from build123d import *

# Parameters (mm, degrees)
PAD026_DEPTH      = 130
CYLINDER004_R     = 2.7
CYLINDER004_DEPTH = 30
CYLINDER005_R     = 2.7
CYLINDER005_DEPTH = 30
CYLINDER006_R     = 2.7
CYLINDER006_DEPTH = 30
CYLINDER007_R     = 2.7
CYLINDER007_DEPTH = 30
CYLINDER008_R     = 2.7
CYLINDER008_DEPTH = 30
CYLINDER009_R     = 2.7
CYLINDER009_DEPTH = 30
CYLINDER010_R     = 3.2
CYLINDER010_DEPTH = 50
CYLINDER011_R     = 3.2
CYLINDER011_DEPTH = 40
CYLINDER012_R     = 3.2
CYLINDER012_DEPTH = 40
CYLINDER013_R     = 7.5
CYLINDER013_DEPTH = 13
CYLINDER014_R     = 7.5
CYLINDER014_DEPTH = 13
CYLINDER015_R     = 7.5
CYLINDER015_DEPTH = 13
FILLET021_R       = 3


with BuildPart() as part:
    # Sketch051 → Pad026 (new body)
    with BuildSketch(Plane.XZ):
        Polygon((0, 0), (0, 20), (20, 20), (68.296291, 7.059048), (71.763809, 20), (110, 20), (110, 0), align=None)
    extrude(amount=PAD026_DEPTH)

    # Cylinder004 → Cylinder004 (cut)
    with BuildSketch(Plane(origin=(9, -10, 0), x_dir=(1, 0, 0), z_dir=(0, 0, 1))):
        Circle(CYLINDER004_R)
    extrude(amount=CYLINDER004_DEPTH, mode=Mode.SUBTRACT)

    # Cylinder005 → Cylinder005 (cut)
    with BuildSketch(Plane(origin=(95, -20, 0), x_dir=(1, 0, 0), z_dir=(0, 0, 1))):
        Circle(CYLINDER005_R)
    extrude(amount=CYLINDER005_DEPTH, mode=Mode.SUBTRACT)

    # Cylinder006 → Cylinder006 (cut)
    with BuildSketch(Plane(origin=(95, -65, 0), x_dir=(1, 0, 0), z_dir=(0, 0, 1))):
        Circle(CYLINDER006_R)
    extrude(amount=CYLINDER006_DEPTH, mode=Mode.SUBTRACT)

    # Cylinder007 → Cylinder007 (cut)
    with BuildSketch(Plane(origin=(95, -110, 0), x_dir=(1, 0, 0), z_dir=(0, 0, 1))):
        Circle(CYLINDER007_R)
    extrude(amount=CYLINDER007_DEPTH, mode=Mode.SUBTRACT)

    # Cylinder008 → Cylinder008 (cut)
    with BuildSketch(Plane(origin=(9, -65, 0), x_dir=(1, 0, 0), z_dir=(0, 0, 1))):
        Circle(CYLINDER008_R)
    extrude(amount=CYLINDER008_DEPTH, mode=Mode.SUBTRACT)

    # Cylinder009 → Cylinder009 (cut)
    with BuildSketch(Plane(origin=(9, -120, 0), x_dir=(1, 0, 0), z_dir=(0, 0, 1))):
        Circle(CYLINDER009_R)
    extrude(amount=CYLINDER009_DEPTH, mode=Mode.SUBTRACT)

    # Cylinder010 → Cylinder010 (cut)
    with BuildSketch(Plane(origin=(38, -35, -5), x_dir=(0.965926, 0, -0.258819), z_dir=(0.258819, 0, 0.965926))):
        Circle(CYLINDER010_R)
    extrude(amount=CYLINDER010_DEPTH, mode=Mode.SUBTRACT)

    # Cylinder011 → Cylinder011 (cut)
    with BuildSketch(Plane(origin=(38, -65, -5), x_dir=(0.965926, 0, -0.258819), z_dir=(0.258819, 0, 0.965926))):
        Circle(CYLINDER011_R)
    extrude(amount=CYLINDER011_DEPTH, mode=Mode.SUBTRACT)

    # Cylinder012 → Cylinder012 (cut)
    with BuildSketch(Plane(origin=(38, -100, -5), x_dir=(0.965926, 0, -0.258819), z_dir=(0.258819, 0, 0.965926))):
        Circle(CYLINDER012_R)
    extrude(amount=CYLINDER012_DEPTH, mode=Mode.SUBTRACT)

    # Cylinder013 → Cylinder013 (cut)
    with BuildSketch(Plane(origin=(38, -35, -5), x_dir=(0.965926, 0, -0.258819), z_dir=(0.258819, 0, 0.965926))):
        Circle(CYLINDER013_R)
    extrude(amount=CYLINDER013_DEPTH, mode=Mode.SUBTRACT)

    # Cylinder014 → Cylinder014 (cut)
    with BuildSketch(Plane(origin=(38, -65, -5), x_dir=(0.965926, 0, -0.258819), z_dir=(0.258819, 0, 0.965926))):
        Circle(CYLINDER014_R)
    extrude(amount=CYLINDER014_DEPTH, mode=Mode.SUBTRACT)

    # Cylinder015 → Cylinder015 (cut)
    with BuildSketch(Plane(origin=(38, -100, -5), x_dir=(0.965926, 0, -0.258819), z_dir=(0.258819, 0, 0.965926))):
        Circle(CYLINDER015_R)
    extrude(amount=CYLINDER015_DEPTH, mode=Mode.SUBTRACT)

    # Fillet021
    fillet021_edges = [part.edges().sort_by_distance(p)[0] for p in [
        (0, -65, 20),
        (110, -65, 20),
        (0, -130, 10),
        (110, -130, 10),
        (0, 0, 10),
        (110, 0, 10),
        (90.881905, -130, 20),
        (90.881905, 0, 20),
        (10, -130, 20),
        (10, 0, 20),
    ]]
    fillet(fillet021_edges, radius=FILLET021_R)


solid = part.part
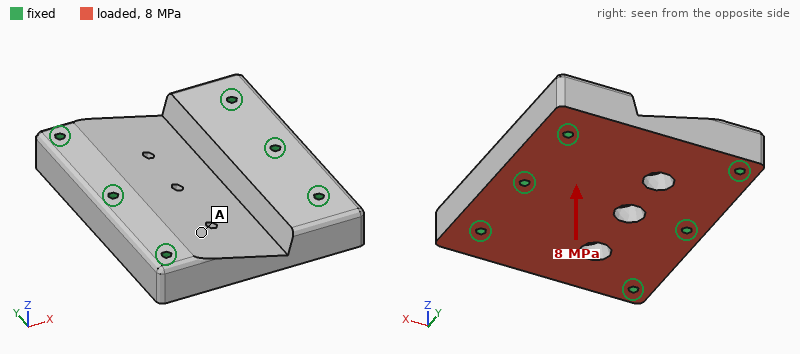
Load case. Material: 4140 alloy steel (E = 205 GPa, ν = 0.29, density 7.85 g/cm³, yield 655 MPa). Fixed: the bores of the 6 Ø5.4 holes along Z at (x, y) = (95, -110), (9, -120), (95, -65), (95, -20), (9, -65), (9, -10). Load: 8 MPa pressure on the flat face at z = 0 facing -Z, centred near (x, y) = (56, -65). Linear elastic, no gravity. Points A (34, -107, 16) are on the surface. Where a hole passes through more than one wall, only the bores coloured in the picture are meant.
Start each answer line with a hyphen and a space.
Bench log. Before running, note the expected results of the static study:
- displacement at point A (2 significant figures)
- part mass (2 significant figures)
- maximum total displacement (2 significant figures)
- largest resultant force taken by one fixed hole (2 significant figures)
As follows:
- 22 µm
- 1.8 kg
- 31 µm
- 22 kN
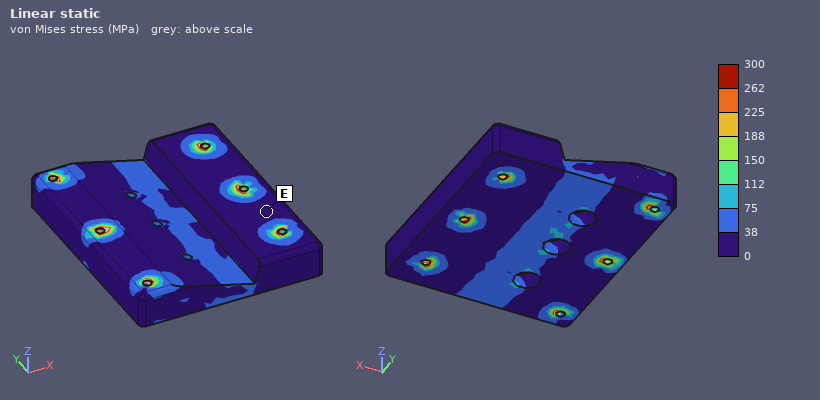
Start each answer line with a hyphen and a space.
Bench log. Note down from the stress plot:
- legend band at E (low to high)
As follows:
- 0 to 38 MPa
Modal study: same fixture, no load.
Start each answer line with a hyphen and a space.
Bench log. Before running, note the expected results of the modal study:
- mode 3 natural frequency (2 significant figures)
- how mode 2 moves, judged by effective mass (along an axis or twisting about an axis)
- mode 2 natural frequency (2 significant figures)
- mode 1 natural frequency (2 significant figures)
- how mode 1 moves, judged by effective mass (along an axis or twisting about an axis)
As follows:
- 13 kHz
- twisting about X
- 10 kHz
- 9000 Hz
- along Z
